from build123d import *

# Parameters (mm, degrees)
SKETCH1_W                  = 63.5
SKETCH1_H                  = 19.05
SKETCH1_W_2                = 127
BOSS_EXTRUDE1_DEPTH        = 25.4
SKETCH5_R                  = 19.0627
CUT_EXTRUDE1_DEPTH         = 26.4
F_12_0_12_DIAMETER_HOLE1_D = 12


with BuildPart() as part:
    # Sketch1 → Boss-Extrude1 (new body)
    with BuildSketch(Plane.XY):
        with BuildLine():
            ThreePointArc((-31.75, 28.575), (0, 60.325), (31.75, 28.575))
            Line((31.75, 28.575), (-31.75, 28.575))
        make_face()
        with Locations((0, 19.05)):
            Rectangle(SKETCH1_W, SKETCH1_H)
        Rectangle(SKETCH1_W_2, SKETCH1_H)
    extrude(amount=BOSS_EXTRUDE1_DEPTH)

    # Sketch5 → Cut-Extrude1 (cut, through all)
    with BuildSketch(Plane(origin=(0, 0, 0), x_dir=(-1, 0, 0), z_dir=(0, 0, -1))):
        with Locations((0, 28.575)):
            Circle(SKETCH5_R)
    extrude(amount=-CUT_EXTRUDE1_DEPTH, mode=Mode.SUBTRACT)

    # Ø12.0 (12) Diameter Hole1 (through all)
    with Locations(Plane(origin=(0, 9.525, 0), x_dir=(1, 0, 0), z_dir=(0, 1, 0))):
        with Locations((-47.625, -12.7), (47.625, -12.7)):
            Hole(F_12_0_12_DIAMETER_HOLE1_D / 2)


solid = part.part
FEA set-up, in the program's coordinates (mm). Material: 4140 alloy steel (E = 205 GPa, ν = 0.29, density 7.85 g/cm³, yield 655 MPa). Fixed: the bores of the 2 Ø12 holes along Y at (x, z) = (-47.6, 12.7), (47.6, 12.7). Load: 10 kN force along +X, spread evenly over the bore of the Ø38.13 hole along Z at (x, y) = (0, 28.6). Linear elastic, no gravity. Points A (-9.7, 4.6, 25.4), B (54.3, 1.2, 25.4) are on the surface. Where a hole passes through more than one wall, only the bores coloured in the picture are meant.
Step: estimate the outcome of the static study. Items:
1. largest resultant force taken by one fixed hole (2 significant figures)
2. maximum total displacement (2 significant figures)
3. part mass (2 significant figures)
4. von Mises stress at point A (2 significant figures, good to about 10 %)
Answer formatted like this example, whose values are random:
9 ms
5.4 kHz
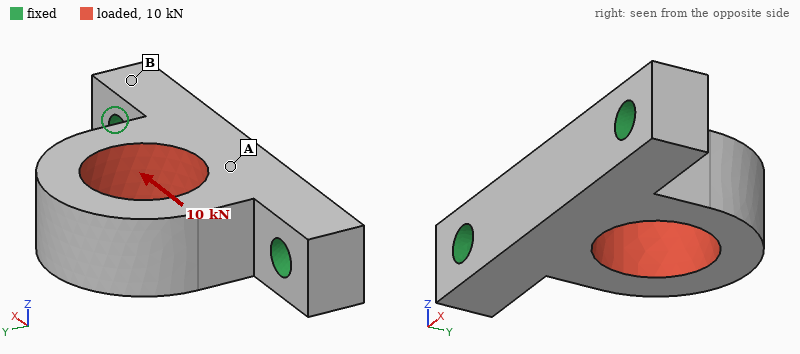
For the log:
6.2 kN
19 µm
780 g
14 MPa
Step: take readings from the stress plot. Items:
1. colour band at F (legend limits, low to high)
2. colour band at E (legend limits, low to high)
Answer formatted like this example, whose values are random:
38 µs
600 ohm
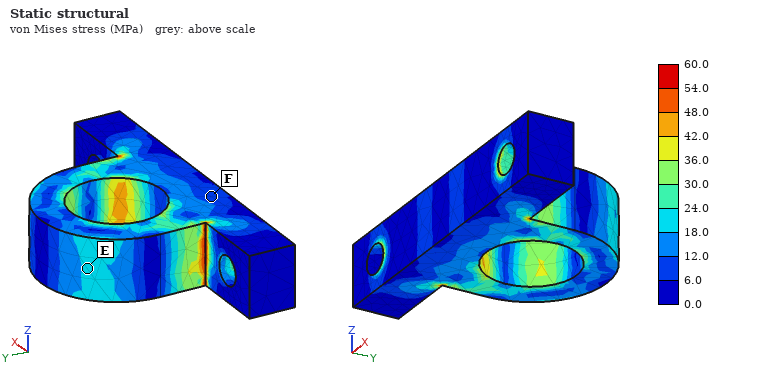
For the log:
6.0 to 12.0 MPa
18.0 to 24.0 MPa
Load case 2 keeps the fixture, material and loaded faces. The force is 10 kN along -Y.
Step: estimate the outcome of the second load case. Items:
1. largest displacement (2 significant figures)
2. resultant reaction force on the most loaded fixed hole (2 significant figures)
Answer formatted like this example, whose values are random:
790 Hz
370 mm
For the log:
7.1 µm
5.2 kN
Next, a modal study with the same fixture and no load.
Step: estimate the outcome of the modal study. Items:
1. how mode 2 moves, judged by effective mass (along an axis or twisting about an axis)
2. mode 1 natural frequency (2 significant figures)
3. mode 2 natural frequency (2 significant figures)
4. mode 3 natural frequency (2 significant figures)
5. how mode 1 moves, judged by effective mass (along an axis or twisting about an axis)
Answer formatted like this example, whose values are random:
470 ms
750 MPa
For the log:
along X
3200 Hz
6300 Hz
8400 Hz
along Z
